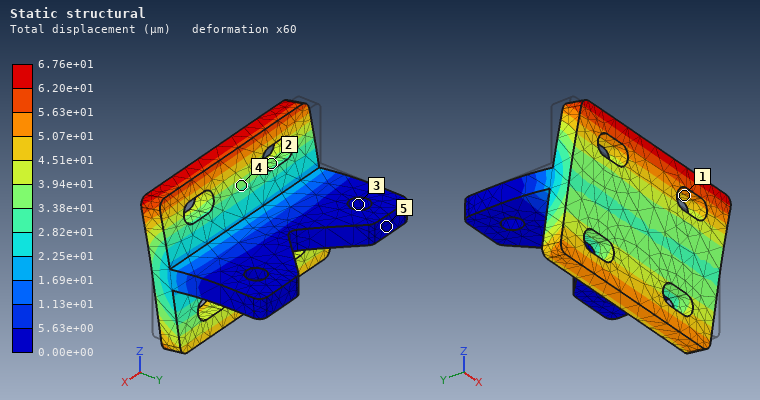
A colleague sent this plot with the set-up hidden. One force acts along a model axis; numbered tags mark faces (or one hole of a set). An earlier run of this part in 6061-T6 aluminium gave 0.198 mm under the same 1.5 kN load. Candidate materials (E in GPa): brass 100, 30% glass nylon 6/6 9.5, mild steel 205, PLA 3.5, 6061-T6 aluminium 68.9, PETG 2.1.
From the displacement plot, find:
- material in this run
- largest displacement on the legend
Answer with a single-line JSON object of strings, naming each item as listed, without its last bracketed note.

{"material in this run": "mild steel", "largest displacement on the legend": "6.76e+01 µm"}
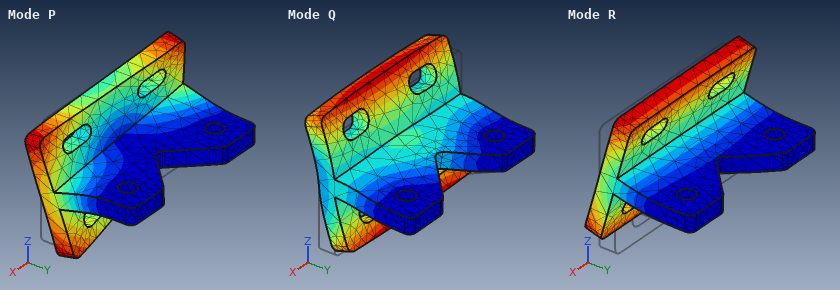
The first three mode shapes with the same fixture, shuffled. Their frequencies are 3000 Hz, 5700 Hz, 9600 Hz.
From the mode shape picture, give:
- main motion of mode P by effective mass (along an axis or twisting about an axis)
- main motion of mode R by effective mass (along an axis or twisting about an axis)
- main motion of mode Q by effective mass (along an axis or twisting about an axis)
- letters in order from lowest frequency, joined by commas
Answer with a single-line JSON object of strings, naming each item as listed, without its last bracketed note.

{"main motion of mode P by effective mass": "twisting about Y", "main motion of mode R by effective mass": "along Z", "main motion of mode Q by effective mass": "along Z", "letters in order from lowest frequency, joined by commas": "R, P, Q"}
